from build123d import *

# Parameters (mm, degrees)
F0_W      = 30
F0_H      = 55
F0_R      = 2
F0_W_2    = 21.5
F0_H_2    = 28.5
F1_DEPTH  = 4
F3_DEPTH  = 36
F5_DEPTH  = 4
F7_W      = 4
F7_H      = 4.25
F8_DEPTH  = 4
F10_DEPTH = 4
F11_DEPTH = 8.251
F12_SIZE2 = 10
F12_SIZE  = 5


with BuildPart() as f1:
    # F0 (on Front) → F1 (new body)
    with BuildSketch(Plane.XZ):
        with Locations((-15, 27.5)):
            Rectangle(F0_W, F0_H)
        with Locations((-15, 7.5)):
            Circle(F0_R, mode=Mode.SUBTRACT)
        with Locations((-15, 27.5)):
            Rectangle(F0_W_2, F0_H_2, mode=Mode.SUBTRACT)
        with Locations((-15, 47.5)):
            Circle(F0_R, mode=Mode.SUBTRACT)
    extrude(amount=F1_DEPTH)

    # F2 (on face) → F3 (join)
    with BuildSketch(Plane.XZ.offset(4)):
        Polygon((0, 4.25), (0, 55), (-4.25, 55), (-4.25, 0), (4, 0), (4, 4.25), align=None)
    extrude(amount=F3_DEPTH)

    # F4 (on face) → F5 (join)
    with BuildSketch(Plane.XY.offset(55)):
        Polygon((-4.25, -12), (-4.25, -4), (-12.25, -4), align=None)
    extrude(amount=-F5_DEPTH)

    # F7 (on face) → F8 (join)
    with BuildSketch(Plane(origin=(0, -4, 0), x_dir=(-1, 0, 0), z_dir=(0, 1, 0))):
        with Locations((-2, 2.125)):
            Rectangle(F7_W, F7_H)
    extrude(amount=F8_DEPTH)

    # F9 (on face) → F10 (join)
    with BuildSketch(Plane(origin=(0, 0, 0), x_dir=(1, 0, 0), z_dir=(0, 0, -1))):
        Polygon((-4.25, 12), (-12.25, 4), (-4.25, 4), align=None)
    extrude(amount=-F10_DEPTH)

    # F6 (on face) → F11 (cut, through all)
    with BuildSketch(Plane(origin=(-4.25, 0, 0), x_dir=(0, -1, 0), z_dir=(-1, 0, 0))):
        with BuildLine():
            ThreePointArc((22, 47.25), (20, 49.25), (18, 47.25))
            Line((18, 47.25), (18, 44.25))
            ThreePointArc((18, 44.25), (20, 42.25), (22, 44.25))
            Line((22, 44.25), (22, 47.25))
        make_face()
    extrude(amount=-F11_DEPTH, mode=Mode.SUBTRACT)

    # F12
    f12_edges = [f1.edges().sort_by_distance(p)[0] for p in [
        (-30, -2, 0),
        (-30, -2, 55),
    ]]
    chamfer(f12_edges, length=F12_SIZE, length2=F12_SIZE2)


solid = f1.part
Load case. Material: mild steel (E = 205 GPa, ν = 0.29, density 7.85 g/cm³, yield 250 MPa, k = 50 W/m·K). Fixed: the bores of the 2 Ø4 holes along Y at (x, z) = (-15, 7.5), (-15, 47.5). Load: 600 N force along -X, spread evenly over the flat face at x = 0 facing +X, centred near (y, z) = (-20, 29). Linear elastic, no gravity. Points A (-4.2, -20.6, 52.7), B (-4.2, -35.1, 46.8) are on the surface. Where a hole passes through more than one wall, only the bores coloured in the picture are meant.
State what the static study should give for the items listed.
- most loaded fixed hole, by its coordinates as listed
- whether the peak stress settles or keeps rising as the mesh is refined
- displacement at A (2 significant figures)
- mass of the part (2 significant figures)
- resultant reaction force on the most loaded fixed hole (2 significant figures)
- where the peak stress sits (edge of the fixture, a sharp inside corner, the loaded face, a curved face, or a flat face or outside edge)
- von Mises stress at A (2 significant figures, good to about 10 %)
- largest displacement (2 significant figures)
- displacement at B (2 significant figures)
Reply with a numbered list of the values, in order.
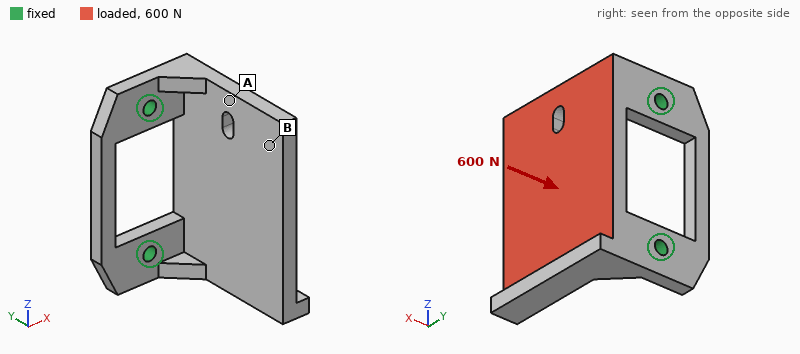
1. (-15, 47.5)
2. keeps rising
3. 0.058 mm
4. 100 g
5. 350 N
6. edge of the fixture
7. 29 MPa
8. 0.15 mm
9. 0.12 mm
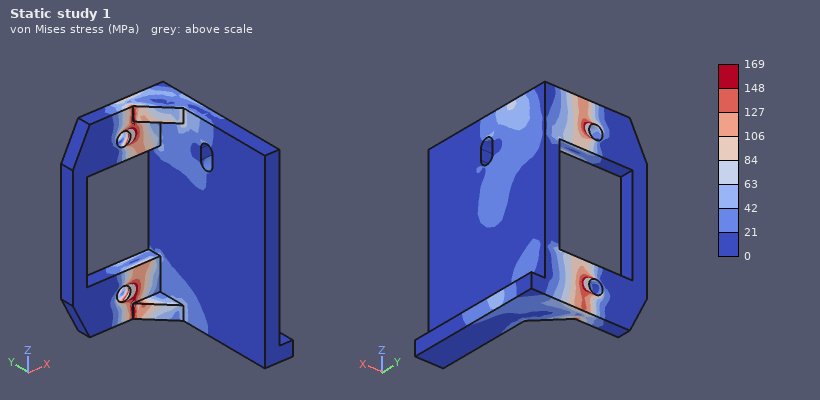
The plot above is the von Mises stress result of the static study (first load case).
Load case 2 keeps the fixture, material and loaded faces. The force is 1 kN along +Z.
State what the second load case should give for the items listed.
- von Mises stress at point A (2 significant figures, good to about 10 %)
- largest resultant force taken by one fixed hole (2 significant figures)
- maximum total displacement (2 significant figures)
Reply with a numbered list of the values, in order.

1. 18 MPa
2. 660 N
3. 26 µm
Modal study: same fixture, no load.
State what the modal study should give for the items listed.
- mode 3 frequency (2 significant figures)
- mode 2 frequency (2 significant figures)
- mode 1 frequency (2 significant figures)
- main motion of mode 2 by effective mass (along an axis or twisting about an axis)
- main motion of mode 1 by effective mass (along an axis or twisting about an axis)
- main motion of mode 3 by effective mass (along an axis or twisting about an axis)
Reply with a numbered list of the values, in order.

1. 5400 Hz
2. 3200 Hz
3. 1400 Hz
4. along Z
5. along X
6. along Z
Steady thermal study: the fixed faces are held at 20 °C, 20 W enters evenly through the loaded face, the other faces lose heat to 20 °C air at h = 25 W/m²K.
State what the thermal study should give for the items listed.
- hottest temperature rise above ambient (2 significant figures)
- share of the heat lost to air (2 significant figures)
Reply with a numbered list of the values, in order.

1. 60 K
2. 23 %
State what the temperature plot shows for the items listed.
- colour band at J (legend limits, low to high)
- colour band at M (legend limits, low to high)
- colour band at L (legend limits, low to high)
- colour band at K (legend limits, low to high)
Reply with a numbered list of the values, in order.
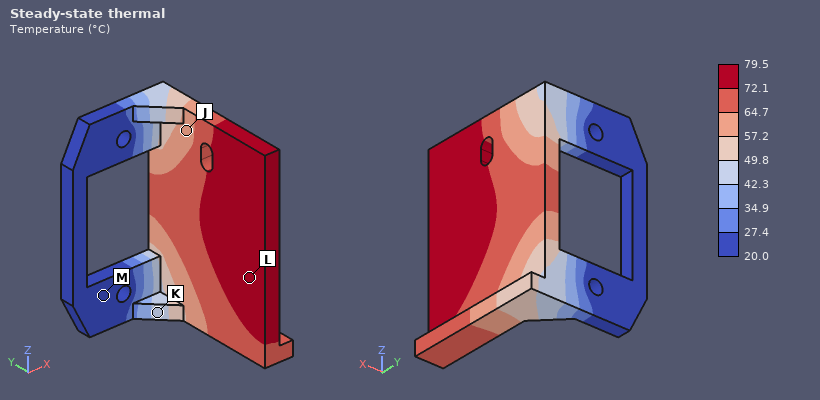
1. 57.2 to 64.7 °C
2. 20.0 to 27.4 °C
3. 72.1 to 79.5 °C
4. 42.3 to 49.8 °C
